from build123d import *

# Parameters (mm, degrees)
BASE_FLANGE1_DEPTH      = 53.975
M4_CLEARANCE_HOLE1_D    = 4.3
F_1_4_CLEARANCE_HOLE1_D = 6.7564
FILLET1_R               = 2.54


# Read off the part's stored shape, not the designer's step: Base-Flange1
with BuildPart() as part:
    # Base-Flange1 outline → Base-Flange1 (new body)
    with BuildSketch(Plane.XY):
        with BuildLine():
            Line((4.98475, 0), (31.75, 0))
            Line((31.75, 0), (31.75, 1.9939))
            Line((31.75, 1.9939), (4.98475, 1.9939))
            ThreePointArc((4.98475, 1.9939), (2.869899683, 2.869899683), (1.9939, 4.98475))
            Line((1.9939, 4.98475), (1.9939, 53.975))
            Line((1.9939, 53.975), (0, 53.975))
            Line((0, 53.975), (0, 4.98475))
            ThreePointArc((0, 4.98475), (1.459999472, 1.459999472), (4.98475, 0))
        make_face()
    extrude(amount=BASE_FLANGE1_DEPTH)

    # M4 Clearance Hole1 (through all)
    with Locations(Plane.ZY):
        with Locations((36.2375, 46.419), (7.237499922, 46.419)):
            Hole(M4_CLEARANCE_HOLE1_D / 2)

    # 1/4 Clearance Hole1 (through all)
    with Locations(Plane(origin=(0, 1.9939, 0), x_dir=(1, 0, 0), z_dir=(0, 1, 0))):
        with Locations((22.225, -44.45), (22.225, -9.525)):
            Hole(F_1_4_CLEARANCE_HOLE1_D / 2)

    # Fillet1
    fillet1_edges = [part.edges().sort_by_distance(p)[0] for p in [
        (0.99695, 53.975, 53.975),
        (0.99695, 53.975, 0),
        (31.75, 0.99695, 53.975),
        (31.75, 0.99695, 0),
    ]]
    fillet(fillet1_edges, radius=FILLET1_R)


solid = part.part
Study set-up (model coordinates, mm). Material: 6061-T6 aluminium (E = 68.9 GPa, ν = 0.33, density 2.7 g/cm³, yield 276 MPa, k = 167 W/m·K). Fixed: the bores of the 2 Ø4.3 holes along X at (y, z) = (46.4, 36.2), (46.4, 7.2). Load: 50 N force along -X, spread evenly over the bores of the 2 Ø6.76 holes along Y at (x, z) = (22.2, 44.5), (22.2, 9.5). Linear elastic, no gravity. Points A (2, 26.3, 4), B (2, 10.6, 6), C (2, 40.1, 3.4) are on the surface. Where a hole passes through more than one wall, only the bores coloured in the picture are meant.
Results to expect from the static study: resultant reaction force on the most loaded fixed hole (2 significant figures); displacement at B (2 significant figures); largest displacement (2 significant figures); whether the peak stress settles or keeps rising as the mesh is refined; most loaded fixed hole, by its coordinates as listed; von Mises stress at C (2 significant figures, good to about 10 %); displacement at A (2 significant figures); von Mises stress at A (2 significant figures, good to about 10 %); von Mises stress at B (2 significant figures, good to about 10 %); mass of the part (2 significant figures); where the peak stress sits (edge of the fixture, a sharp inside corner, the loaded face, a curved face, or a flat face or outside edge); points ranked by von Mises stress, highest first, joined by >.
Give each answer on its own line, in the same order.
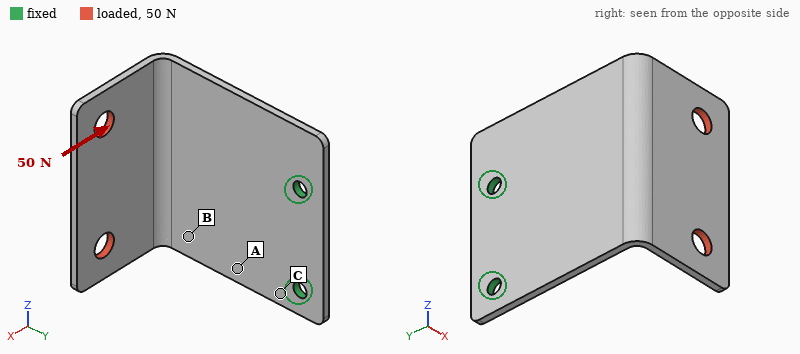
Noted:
34 N
0.42 mm
0.91 mm
keeps rising
(46.4, 36.2)
60 MPa
0.15 mm
36 MPa
14 MPa
23 g
edge of the fixture
C > A > B
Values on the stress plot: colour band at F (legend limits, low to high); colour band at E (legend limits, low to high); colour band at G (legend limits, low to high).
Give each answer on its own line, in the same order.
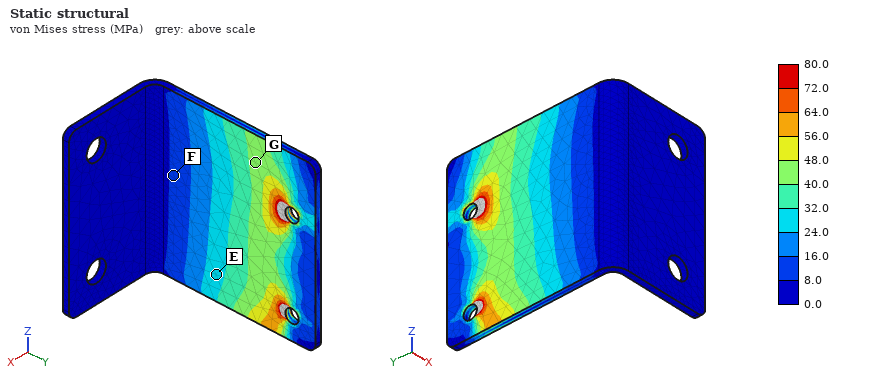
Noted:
8.0 to 16.0 MPa
24.0 to 32.0 MPa
40.0 to 48.0 MPa
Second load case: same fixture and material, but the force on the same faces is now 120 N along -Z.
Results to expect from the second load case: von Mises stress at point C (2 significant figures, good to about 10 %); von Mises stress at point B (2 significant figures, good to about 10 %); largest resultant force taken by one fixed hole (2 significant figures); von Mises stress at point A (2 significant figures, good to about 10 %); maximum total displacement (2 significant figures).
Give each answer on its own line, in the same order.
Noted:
52 MPa
51 MPa
200 N
50 MPa
0.82 mm
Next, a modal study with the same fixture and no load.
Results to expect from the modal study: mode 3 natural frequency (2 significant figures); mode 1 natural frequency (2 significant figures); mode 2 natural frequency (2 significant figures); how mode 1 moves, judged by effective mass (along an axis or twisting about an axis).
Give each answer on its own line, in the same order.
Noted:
1300 Hz
380 Hz
760 Hz
along X
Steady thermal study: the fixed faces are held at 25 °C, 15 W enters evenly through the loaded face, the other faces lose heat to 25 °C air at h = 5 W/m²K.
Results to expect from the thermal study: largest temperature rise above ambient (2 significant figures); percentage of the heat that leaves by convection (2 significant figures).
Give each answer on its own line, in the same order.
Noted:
59 K
8.7 %
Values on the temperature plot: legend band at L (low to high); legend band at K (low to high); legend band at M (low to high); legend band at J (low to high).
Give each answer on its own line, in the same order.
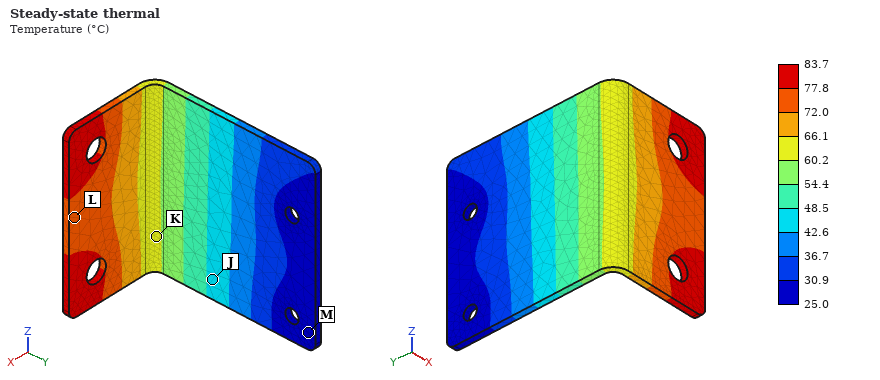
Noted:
72.0 to 77.8 °C
60.2 to 66.1 °C
25.0 to 30.9 °C
42.6 to 48.5 °C
